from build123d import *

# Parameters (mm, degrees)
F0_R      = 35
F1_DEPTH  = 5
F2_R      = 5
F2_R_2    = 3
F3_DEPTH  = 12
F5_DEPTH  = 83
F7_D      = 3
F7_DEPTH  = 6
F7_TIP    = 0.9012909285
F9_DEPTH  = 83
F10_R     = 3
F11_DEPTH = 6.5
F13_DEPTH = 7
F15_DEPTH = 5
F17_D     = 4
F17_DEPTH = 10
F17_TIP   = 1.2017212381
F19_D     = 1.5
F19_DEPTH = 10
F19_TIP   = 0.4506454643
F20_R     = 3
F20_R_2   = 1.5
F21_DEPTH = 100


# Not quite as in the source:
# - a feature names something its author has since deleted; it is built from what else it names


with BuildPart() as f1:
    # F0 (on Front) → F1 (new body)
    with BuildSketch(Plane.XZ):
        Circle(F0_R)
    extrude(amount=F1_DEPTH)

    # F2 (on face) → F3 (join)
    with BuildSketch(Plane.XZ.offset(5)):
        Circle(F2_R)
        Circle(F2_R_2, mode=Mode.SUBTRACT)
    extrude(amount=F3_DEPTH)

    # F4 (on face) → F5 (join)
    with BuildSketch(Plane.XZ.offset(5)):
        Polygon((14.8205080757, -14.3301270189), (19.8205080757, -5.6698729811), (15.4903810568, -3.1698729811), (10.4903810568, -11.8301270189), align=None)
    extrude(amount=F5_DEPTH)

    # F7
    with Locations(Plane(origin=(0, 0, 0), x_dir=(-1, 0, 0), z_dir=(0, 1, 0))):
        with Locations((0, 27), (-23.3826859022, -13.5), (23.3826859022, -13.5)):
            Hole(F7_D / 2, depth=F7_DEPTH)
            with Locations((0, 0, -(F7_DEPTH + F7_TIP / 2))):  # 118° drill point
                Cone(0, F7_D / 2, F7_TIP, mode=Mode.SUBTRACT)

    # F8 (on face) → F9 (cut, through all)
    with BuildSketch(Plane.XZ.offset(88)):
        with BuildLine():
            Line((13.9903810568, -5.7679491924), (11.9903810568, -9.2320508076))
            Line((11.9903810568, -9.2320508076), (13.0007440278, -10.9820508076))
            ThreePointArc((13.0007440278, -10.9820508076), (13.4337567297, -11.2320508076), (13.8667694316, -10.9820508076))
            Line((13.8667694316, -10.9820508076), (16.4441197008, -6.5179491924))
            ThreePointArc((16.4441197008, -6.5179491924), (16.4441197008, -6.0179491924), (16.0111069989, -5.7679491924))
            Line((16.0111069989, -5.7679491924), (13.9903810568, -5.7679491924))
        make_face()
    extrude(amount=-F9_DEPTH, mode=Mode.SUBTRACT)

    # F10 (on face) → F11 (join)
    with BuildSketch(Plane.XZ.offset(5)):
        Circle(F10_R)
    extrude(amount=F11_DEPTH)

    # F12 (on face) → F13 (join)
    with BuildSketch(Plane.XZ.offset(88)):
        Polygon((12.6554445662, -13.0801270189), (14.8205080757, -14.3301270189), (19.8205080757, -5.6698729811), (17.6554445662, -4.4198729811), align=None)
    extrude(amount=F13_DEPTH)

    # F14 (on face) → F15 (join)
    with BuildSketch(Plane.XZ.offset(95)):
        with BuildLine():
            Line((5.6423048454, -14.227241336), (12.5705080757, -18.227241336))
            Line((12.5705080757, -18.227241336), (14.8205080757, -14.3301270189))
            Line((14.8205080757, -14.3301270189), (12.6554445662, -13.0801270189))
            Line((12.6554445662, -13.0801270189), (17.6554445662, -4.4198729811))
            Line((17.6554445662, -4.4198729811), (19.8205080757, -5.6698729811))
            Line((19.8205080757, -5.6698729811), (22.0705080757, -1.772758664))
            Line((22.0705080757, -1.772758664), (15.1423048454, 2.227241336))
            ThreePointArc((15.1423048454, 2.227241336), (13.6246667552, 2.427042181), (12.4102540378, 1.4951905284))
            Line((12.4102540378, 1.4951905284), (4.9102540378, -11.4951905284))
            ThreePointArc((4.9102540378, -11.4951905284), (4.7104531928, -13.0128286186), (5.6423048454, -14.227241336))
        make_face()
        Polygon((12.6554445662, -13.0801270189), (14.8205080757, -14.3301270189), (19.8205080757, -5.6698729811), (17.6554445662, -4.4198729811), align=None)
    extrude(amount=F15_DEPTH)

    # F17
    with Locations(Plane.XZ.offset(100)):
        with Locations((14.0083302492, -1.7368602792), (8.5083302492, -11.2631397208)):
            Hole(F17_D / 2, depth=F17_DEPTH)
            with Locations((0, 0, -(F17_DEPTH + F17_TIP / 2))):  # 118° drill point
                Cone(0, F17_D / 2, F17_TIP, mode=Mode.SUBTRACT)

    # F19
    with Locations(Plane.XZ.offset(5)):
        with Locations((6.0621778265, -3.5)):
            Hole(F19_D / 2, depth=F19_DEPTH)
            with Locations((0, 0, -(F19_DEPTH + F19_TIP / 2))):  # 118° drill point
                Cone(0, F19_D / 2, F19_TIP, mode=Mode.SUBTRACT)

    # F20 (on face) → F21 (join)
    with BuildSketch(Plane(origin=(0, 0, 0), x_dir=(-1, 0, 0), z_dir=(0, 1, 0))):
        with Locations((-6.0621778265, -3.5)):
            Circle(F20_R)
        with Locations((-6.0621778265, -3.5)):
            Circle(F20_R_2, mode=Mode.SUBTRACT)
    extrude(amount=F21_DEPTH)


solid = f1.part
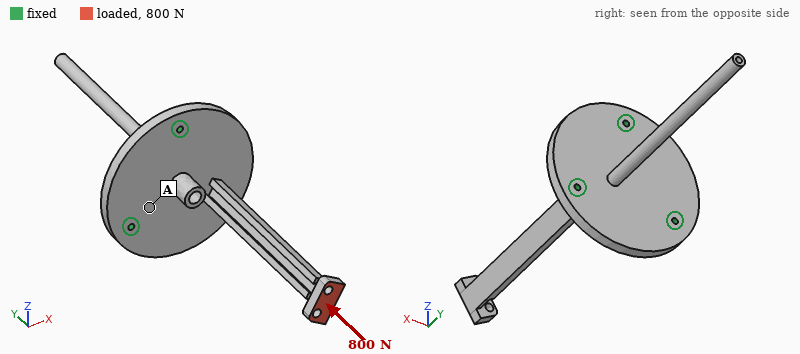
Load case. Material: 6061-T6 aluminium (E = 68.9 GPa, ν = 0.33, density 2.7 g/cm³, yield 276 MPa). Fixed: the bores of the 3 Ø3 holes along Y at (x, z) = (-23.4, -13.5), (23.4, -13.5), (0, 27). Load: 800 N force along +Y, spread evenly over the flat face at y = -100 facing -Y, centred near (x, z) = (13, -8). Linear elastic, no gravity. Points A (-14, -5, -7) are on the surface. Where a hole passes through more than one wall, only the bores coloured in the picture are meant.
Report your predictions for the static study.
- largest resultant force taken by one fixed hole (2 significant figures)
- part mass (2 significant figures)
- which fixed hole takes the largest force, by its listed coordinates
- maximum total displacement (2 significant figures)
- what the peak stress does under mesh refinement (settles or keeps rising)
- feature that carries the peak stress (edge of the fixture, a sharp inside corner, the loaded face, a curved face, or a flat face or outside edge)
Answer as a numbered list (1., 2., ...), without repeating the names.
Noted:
1. 600 N
2. 70 g
3. (23.4, -13.5)
4. 2.3 mm
5. keeps rising
6. a sharp inside corner
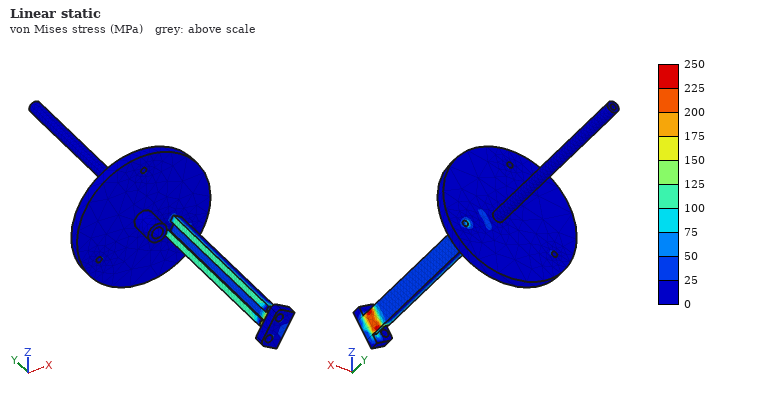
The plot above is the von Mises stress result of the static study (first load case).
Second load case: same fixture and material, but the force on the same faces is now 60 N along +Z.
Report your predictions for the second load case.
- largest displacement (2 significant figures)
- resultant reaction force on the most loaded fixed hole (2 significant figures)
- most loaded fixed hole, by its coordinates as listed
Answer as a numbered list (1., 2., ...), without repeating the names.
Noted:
1. 2.1 mm
2. 100 N
3. (0, 27)
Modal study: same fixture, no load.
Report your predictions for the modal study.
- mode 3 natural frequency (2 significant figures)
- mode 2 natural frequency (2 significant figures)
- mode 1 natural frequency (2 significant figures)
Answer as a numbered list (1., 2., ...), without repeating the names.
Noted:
1. 460 Hz
2. 450 Hz
3. 340 Hz
